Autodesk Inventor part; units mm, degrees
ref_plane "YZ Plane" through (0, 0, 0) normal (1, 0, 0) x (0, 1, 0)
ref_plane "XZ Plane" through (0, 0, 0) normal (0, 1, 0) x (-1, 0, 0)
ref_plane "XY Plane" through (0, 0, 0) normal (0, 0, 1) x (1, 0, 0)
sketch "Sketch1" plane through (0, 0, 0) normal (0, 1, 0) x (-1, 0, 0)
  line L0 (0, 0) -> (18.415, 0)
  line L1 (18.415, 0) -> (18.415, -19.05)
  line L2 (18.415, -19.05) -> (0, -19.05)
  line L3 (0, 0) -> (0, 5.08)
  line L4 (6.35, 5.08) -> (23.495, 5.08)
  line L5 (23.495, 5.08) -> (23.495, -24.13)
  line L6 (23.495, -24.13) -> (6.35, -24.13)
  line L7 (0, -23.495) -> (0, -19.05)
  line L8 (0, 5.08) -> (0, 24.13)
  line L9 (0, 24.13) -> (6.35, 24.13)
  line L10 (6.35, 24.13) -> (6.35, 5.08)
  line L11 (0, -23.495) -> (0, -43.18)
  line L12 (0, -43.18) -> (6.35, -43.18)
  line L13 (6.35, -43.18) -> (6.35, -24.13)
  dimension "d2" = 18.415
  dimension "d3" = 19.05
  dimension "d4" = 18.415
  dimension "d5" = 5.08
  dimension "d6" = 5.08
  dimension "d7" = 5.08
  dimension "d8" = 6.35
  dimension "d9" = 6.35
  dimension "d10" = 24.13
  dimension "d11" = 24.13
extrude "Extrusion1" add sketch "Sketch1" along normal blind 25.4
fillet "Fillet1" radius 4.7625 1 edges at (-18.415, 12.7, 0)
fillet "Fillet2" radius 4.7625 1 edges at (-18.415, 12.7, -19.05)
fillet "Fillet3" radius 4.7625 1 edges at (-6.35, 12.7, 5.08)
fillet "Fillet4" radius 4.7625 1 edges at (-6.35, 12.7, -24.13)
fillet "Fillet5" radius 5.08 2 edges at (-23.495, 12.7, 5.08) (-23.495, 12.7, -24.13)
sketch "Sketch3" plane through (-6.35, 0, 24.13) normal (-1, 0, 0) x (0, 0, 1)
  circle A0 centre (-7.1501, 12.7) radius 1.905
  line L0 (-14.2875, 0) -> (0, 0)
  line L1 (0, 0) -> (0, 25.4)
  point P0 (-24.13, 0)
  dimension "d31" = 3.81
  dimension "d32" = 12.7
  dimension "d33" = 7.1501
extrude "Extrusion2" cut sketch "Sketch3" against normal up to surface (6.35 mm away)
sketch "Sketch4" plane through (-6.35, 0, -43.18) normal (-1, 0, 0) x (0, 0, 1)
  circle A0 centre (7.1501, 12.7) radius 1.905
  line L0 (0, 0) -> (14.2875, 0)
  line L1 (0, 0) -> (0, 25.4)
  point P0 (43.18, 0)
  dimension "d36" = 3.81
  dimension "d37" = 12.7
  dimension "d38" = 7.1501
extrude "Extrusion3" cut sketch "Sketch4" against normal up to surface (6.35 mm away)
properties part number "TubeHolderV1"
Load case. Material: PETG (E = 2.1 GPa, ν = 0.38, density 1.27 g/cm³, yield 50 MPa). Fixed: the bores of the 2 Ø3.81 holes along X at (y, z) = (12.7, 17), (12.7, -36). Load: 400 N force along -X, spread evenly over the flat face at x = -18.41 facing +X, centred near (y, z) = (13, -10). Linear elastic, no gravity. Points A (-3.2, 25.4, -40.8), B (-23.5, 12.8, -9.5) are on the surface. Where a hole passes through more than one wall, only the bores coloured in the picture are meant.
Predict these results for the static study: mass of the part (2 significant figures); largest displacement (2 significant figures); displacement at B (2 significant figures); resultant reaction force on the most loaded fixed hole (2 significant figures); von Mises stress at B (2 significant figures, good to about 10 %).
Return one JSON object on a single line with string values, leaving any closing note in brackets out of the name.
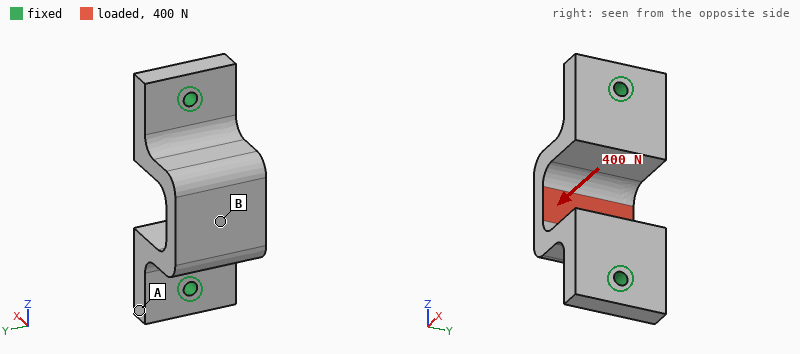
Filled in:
{"mass of the part": "19 g", "largest displacement": "0.15 mm", "displacement at B": "0.13 mm", "resultant reaction force on the most loaded fixed hole": "260 N", "von Mises stress at B": "6.0 MPa"}
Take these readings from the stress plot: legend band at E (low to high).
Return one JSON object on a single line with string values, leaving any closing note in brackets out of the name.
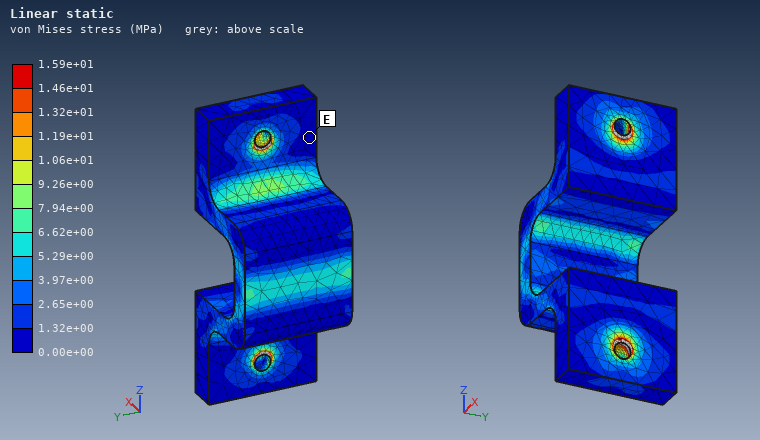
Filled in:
{"legend band at E": "0.00e+00 to 1.32e+00 MPa"}
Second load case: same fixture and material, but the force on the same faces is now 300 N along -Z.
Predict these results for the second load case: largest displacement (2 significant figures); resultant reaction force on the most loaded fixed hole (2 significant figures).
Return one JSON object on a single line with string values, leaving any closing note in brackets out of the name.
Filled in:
{"largest displacement": "0.13 mm", "resultant reaction force on the most loaded fixed hole": "170 N"}
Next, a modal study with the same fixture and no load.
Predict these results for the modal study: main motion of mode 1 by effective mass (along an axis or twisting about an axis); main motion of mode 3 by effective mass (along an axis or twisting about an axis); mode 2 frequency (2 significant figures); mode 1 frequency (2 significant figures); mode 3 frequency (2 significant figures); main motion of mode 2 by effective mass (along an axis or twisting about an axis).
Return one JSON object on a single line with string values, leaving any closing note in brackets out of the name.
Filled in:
{"main motion of mode 1 by effective mass": "along Y", "main motion of mode 3 by effective mass": "along Z", "mode 2 frequency": "2700 Hz", "mode 1 frequency": "1300 Hz", "mode 3 frequency": "2900 Hz", "main motion of mode 2 by effective mass": "along X"}
